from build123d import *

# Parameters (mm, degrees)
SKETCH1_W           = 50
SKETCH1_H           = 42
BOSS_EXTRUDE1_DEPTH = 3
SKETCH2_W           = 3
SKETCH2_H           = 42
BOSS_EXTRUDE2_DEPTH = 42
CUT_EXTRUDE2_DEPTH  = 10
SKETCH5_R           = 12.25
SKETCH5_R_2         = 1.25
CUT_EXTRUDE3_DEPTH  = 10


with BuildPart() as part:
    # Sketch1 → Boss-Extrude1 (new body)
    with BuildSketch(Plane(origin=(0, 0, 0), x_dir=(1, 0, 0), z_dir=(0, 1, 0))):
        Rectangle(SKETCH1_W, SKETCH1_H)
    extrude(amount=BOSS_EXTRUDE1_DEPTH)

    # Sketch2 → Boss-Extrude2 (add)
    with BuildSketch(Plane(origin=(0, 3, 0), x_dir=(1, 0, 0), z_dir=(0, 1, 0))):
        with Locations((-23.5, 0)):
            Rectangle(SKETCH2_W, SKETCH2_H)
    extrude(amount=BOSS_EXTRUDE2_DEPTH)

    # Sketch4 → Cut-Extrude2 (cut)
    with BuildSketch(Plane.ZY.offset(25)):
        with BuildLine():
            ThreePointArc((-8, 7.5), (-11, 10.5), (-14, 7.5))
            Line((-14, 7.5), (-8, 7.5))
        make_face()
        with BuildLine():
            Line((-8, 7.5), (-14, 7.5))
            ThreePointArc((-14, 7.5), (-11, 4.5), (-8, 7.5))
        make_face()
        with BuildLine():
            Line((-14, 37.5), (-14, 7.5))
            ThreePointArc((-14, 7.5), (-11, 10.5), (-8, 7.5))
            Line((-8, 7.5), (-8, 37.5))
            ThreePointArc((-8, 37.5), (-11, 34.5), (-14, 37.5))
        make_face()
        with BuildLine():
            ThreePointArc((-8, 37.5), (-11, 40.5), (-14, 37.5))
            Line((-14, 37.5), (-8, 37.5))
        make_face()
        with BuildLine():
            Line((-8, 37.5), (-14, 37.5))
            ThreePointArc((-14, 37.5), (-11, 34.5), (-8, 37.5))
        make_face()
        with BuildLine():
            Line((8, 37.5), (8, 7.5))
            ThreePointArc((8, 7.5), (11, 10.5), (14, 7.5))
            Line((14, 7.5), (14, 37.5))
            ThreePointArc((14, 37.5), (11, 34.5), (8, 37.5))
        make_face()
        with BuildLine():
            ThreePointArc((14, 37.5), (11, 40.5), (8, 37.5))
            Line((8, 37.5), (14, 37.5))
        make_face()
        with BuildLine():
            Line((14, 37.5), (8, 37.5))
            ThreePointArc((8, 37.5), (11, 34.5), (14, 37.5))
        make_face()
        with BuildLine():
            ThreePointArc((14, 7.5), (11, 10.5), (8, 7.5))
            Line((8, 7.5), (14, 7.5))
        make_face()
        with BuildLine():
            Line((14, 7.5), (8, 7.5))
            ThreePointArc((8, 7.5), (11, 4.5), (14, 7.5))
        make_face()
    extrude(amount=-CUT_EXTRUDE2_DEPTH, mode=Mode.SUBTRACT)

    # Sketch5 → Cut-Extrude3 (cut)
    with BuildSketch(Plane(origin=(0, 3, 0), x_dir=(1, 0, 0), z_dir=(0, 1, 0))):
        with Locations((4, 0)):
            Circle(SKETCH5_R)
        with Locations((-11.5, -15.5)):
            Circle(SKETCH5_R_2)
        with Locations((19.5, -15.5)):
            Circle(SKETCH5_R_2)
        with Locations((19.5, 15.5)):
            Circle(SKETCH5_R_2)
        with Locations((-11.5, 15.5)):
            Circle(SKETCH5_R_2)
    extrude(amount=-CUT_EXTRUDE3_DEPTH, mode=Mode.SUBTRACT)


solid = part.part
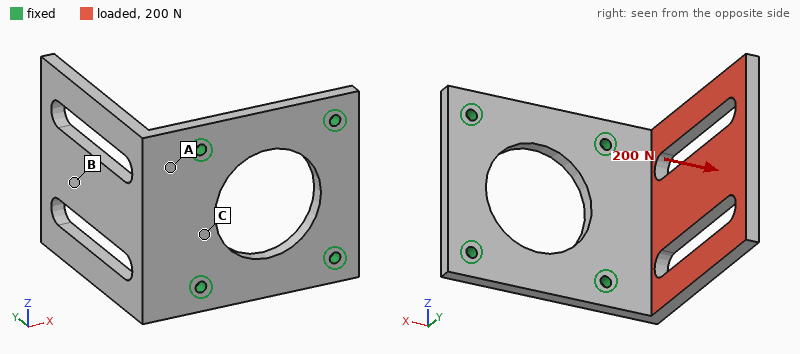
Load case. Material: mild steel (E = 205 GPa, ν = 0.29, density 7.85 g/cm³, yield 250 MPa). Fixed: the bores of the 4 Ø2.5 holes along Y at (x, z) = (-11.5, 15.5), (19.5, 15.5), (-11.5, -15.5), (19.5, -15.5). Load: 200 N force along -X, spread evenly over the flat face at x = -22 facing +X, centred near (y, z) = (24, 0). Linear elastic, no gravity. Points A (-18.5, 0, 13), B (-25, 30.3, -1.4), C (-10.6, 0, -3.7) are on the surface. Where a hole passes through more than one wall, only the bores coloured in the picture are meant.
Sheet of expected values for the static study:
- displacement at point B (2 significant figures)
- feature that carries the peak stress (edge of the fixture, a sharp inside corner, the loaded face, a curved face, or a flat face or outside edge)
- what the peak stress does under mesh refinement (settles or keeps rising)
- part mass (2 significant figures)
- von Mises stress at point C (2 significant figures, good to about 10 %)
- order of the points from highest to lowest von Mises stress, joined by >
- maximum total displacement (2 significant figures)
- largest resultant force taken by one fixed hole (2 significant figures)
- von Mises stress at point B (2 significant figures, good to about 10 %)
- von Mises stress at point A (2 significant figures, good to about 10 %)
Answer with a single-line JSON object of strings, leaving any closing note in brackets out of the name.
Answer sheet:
{"displacement at point B": "0.17 mm", "feature that carries the peak stress": "edge of the fixture", "what the peak stress does under mesh refinement": "keeps rising", "part mass": "70 g", "von Mises stress at point C": "31 MPa", "order of the points from highest to lowest von Mises stress, joined by >": "A > C > B", "maximum total displacement": "0.28 mm", "largest resultant force taken by one fixed hole": "100 N", "von Mises stress at point B": "13 MPa", "von Mises stress at point A": "66 MPa"}
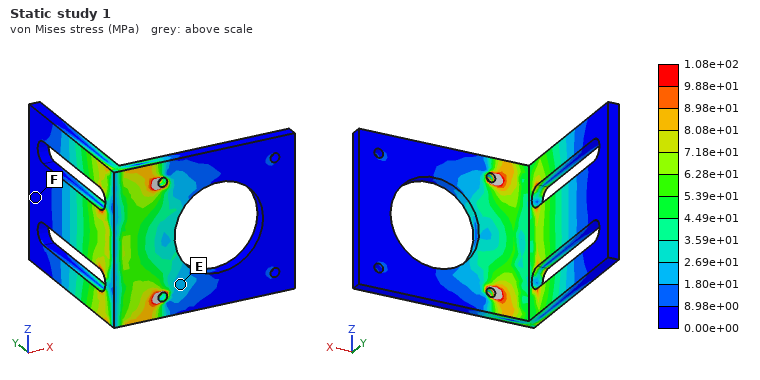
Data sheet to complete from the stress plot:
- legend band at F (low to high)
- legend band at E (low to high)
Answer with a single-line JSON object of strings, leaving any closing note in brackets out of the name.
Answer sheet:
{"legend band at F": "0.00e+00 to 8.98e+00 MPa", "legend band at E": "1.80e+01 to 2.69e+01 MPa"}
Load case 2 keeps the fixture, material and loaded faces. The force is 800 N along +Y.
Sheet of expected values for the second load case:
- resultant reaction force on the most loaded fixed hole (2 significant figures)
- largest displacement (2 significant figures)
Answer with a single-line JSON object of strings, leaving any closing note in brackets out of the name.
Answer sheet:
{"resultant reaction force on the most loaded fixed hole": "420 N", "largest displacement": "86 µm"}
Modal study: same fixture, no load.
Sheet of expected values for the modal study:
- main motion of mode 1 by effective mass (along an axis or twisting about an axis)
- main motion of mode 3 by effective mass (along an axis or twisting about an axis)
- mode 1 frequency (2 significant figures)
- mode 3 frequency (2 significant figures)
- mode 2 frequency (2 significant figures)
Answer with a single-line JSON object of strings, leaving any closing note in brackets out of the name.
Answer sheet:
{"main motion of mode 1 by effective mass": "along X", "main motion of mode 3 by effective mass": "along Z", "mode 1 frequency": "910 Hz", "mode 3 frequency": "3200 Hz", "mode 2 frequency": "2400 Hz"}
